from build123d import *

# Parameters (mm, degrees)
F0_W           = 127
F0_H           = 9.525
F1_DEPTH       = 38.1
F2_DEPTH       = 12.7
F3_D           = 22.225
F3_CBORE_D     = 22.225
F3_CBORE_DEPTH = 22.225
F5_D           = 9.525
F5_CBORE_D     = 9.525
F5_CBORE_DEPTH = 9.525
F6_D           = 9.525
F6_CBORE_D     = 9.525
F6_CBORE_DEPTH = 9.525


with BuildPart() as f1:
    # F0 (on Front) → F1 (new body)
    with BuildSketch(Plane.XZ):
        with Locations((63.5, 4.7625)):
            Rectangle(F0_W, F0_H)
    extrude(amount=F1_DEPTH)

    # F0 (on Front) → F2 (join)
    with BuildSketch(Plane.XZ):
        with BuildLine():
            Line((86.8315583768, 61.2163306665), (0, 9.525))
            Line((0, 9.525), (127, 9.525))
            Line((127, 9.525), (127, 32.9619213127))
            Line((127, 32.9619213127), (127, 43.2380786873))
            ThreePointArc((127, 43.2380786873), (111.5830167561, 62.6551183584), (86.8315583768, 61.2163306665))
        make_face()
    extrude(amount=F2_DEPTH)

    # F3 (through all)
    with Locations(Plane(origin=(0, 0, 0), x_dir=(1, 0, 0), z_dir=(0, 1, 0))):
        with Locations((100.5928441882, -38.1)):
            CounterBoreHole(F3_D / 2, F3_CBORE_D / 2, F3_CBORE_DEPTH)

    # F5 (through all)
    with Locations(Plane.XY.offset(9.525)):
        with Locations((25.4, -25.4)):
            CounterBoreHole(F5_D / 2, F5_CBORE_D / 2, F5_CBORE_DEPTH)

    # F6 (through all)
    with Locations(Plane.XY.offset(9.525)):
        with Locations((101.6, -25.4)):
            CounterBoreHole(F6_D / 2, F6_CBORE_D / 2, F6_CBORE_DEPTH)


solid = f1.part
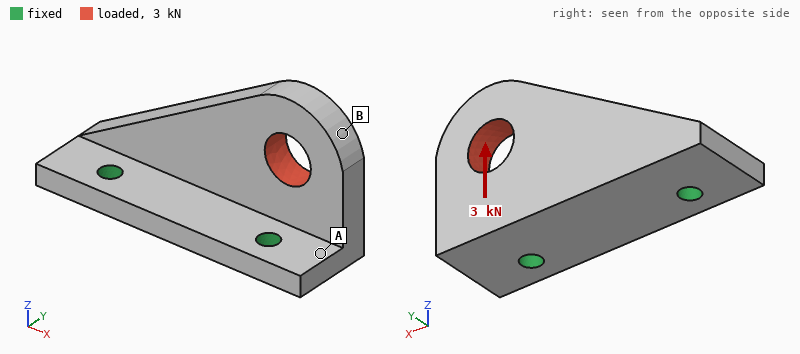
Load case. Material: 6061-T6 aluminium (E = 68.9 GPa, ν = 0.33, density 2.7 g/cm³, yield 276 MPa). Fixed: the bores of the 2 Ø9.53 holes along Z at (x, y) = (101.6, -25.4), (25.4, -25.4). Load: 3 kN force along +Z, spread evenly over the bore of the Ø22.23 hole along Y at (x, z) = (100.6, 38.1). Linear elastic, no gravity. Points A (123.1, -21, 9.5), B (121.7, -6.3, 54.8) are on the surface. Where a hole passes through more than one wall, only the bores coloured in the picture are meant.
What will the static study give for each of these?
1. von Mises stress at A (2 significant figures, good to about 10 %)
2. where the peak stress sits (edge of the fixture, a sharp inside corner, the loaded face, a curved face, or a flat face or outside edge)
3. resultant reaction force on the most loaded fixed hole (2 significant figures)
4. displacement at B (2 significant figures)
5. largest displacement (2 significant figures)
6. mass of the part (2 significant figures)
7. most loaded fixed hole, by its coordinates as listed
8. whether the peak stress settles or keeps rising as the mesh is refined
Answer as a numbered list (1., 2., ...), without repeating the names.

1. 16 MPa
2. edge of the fixture
3. 2.9 kN
4. 87 µm
5. 98 µm
6. 260 g
7. (101.6, -25.4)
8. keeps rising
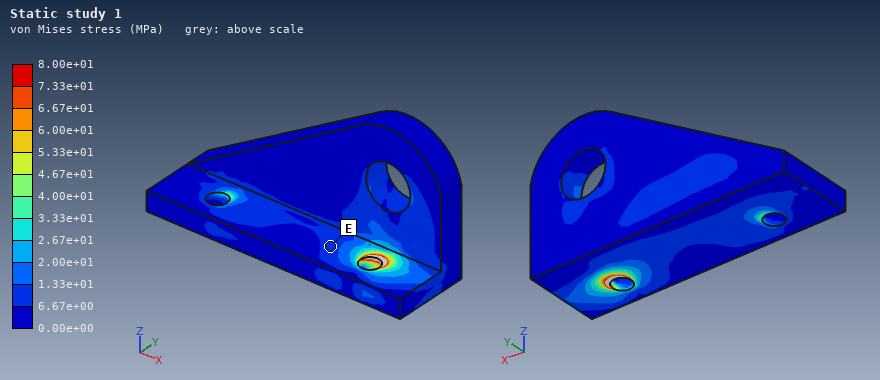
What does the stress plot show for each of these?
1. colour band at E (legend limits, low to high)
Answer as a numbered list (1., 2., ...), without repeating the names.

1. 6.67e+00 to 1.33e+01 MPa
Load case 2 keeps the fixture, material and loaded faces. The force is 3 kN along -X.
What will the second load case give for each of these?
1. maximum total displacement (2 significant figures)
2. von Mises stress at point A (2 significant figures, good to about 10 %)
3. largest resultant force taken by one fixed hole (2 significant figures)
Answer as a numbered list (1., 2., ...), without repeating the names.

1. 33 µm
2. 5.6 MPa
3. 2.1 kN
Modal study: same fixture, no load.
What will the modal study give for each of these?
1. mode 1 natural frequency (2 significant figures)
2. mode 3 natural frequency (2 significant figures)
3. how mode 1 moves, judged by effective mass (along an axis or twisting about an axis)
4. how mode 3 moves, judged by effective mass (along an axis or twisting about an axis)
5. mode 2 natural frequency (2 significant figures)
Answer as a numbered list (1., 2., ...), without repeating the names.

1. 2000 Hz
2. 6100 Hz
3. along Y
4. along Z
5. 4800 Hz
